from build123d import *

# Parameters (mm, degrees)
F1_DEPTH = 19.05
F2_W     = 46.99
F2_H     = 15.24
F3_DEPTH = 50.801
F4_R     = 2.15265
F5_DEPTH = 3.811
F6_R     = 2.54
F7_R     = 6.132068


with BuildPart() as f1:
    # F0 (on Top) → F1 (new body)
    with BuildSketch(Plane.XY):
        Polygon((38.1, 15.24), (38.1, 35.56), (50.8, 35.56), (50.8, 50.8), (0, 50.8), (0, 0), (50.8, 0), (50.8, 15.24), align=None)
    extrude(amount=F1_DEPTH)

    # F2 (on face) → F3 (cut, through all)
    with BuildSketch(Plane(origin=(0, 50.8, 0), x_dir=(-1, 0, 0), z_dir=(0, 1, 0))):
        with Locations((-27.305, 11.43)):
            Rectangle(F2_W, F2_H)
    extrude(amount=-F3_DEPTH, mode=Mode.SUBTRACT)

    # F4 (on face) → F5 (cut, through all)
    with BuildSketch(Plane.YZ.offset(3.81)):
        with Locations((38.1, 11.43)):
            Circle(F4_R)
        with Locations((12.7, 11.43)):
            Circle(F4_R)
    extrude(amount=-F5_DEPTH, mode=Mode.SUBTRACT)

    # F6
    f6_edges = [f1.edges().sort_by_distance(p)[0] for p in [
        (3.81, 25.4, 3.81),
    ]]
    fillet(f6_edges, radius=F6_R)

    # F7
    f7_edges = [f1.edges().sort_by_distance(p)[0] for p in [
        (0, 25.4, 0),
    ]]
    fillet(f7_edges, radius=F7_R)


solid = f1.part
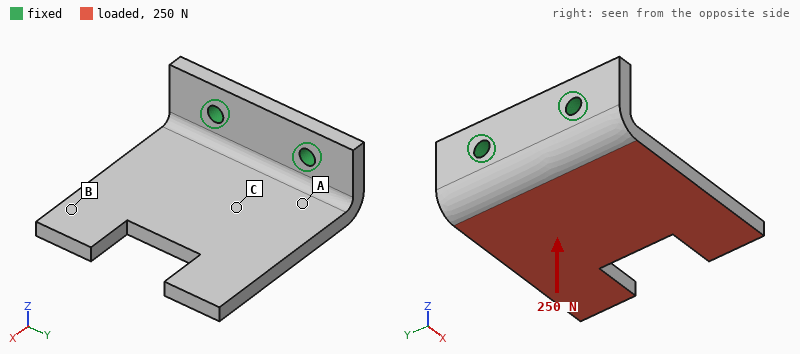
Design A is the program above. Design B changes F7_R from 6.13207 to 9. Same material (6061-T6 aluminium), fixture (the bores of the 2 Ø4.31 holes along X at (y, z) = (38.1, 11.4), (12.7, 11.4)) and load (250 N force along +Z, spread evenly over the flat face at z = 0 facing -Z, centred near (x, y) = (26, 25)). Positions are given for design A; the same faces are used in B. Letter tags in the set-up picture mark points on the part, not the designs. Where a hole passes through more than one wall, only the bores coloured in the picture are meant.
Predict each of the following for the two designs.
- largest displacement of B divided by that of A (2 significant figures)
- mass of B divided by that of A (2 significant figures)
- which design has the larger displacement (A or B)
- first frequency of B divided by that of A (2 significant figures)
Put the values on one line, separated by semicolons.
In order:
1.5; 0.96; B; 0.86
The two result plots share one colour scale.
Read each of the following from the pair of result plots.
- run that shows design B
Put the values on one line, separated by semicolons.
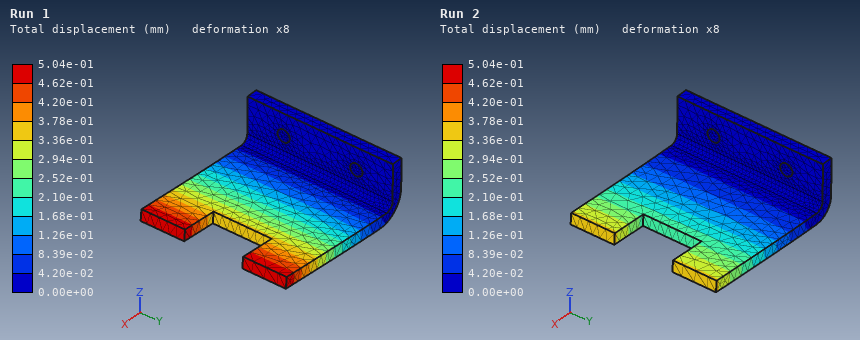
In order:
Run 1
